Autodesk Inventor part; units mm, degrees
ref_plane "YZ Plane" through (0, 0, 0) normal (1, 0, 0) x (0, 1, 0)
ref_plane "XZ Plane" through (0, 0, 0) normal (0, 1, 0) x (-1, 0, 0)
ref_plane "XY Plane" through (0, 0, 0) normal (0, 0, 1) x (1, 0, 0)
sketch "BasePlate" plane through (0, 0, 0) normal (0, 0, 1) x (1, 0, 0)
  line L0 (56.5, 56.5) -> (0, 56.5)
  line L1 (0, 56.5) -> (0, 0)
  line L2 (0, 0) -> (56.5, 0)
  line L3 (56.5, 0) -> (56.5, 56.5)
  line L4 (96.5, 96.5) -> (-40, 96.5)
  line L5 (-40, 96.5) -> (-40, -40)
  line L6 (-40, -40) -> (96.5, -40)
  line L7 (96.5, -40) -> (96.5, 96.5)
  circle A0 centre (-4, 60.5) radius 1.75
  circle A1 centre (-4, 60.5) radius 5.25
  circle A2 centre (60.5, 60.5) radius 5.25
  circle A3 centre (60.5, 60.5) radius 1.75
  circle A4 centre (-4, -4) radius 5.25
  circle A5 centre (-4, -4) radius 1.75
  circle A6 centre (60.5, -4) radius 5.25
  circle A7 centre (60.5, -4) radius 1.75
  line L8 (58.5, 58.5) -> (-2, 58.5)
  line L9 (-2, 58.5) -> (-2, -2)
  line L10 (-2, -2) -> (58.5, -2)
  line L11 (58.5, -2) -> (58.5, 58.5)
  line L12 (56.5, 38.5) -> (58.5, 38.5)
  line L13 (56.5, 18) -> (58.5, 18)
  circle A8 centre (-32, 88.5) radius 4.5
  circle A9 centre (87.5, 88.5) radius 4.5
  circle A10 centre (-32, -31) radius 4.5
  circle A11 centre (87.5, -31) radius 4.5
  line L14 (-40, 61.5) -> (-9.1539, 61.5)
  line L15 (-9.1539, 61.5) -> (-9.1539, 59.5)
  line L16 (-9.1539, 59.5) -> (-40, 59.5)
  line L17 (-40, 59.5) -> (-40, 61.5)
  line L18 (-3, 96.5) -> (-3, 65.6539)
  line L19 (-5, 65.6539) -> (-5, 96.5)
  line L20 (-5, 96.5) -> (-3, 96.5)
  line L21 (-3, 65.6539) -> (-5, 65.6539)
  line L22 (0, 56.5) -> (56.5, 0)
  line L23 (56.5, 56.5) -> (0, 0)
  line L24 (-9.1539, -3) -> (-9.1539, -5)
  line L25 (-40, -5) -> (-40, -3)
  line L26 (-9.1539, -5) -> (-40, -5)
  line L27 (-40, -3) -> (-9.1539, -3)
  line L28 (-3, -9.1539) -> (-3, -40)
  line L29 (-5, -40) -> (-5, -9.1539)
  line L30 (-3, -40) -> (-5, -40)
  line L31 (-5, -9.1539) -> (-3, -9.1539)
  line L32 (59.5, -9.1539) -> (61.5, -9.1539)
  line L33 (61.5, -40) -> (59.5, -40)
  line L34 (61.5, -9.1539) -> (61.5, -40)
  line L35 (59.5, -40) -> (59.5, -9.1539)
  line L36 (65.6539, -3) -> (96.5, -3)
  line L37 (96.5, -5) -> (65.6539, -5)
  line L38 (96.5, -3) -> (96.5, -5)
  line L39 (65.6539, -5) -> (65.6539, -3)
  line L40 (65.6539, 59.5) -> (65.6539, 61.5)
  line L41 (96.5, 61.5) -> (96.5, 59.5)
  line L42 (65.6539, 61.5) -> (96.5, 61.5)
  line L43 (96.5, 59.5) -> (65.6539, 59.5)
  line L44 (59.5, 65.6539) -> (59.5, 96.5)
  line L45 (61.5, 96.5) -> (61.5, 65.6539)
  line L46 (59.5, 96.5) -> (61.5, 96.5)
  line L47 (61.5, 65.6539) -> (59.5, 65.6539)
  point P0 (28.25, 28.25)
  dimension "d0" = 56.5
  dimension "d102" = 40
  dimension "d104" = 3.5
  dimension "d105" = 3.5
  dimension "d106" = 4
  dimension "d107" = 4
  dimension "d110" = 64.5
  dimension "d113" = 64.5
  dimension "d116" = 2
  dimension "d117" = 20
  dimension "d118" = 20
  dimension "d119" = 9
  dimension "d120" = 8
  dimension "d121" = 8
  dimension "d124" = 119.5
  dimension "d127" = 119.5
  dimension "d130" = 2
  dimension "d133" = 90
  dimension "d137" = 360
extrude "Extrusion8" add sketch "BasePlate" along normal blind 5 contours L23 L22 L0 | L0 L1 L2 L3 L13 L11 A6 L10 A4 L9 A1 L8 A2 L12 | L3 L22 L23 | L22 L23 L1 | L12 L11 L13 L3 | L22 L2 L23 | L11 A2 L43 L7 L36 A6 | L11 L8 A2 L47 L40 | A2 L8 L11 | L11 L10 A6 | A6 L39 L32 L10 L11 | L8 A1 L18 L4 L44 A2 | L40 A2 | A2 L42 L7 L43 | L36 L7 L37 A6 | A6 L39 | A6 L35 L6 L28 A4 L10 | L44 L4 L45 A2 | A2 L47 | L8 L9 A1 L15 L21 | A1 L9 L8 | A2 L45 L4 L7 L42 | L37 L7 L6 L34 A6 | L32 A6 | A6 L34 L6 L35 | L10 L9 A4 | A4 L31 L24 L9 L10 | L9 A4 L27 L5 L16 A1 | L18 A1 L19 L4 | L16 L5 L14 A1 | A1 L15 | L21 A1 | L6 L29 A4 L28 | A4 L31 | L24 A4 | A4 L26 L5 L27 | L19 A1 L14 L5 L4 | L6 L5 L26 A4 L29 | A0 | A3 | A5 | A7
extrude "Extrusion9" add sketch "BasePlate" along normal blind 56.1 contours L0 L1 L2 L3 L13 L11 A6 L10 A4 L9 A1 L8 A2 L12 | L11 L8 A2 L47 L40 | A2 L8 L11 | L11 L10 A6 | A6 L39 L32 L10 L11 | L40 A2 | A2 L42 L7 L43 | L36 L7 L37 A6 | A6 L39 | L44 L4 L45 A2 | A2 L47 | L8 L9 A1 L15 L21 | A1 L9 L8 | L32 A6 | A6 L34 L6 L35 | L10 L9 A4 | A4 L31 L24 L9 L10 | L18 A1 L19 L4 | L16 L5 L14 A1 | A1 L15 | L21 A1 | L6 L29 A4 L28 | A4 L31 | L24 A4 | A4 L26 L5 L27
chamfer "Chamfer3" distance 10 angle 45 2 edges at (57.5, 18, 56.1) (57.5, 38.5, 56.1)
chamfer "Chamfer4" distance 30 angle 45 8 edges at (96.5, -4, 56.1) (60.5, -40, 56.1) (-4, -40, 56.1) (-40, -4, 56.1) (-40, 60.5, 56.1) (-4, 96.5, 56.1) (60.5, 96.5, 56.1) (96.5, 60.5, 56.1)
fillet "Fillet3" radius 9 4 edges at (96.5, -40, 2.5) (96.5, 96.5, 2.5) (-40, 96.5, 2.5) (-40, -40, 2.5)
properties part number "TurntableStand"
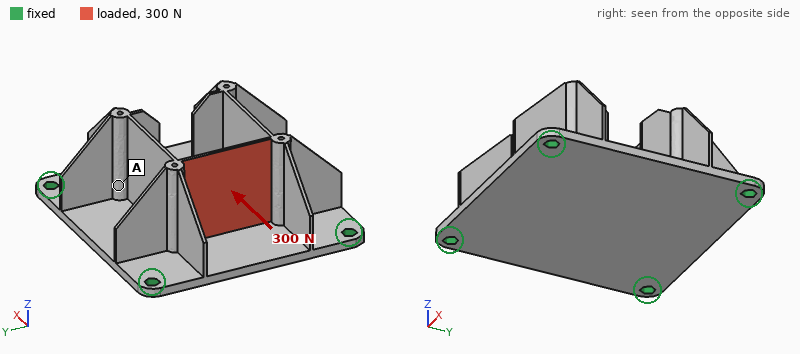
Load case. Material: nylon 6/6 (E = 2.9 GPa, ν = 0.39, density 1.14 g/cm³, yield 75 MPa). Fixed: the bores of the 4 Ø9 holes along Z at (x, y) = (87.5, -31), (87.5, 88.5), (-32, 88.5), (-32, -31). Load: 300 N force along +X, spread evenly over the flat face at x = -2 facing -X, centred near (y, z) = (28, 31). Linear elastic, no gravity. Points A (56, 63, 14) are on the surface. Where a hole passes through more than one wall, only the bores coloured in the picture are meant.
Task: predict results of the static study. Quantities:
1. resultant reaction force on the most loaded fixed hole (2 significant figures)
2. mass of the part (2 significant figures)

96 N
170 g
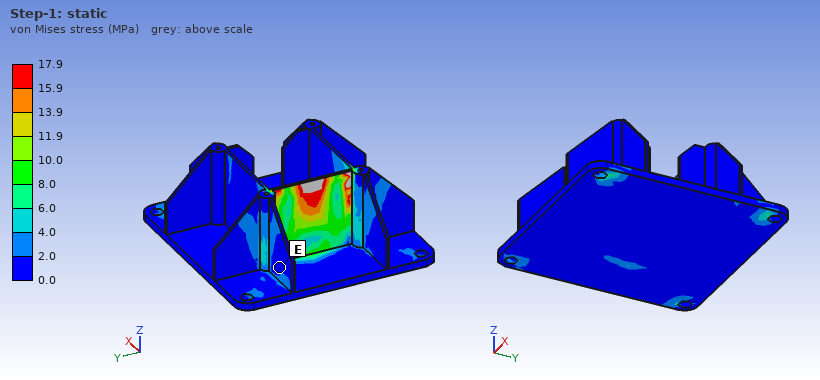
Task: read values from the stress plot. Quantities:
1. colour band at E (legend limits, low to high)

0.0 to 2.0 MPa
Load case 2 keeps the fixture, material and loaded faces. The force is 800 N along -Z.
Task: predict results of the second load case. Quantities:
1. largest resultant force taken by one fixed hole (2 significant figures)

330 N
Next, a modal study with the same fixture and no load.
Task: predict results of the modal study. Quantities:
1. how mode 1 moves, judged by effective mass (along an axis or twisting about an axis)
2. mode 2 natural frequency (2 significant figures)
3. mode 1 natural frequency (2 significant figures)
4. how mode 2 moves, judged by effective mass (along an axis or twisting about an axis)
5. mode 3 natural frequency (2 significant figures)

along Z
640 Hz
450 Hz
along Z
740 Hz
